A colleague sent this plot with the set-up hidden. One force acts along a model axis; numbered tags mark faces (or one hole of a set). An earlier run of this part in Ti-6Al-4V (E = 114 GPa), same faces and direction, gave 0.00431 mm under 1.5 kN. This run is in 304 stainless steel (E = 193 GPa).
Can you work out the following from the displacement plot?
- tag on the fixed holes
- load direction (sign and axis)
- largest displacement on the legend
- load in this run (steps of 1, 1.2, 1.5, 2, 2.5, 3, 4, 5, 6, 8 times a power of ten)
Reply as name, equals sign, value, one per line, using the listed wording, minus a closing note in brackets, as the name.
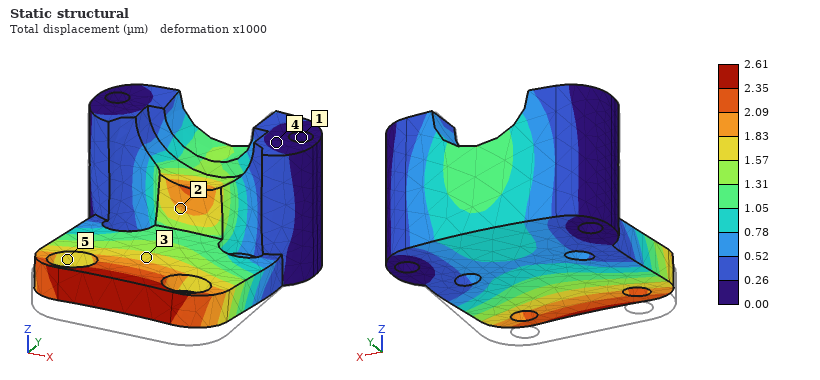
tag on the fixed holes = 1
load direction = +Y
largest displacement on the legend = 2.61 µm
load in this run = 1.5 kN
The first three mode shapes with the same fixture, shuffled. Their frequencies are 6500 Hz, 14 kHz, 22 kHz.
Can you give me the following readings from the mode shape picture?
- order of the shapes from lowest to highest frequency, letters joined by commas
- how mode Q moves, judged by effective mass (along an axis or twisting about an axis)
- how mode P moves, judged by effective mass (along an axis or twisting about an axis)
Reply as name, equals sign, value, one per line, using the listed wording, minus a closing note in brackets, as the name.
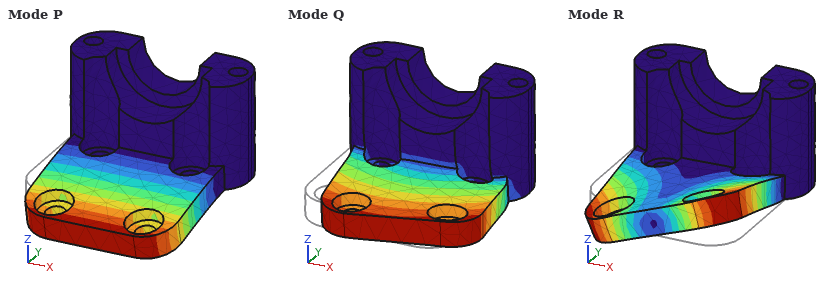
order of the shapes from lowest to highest frequency, letters joined by commas = P, R, Q
how mode Q moves, judged by effective mass = along X
how mode P moves, judged by effective mass = along Z
